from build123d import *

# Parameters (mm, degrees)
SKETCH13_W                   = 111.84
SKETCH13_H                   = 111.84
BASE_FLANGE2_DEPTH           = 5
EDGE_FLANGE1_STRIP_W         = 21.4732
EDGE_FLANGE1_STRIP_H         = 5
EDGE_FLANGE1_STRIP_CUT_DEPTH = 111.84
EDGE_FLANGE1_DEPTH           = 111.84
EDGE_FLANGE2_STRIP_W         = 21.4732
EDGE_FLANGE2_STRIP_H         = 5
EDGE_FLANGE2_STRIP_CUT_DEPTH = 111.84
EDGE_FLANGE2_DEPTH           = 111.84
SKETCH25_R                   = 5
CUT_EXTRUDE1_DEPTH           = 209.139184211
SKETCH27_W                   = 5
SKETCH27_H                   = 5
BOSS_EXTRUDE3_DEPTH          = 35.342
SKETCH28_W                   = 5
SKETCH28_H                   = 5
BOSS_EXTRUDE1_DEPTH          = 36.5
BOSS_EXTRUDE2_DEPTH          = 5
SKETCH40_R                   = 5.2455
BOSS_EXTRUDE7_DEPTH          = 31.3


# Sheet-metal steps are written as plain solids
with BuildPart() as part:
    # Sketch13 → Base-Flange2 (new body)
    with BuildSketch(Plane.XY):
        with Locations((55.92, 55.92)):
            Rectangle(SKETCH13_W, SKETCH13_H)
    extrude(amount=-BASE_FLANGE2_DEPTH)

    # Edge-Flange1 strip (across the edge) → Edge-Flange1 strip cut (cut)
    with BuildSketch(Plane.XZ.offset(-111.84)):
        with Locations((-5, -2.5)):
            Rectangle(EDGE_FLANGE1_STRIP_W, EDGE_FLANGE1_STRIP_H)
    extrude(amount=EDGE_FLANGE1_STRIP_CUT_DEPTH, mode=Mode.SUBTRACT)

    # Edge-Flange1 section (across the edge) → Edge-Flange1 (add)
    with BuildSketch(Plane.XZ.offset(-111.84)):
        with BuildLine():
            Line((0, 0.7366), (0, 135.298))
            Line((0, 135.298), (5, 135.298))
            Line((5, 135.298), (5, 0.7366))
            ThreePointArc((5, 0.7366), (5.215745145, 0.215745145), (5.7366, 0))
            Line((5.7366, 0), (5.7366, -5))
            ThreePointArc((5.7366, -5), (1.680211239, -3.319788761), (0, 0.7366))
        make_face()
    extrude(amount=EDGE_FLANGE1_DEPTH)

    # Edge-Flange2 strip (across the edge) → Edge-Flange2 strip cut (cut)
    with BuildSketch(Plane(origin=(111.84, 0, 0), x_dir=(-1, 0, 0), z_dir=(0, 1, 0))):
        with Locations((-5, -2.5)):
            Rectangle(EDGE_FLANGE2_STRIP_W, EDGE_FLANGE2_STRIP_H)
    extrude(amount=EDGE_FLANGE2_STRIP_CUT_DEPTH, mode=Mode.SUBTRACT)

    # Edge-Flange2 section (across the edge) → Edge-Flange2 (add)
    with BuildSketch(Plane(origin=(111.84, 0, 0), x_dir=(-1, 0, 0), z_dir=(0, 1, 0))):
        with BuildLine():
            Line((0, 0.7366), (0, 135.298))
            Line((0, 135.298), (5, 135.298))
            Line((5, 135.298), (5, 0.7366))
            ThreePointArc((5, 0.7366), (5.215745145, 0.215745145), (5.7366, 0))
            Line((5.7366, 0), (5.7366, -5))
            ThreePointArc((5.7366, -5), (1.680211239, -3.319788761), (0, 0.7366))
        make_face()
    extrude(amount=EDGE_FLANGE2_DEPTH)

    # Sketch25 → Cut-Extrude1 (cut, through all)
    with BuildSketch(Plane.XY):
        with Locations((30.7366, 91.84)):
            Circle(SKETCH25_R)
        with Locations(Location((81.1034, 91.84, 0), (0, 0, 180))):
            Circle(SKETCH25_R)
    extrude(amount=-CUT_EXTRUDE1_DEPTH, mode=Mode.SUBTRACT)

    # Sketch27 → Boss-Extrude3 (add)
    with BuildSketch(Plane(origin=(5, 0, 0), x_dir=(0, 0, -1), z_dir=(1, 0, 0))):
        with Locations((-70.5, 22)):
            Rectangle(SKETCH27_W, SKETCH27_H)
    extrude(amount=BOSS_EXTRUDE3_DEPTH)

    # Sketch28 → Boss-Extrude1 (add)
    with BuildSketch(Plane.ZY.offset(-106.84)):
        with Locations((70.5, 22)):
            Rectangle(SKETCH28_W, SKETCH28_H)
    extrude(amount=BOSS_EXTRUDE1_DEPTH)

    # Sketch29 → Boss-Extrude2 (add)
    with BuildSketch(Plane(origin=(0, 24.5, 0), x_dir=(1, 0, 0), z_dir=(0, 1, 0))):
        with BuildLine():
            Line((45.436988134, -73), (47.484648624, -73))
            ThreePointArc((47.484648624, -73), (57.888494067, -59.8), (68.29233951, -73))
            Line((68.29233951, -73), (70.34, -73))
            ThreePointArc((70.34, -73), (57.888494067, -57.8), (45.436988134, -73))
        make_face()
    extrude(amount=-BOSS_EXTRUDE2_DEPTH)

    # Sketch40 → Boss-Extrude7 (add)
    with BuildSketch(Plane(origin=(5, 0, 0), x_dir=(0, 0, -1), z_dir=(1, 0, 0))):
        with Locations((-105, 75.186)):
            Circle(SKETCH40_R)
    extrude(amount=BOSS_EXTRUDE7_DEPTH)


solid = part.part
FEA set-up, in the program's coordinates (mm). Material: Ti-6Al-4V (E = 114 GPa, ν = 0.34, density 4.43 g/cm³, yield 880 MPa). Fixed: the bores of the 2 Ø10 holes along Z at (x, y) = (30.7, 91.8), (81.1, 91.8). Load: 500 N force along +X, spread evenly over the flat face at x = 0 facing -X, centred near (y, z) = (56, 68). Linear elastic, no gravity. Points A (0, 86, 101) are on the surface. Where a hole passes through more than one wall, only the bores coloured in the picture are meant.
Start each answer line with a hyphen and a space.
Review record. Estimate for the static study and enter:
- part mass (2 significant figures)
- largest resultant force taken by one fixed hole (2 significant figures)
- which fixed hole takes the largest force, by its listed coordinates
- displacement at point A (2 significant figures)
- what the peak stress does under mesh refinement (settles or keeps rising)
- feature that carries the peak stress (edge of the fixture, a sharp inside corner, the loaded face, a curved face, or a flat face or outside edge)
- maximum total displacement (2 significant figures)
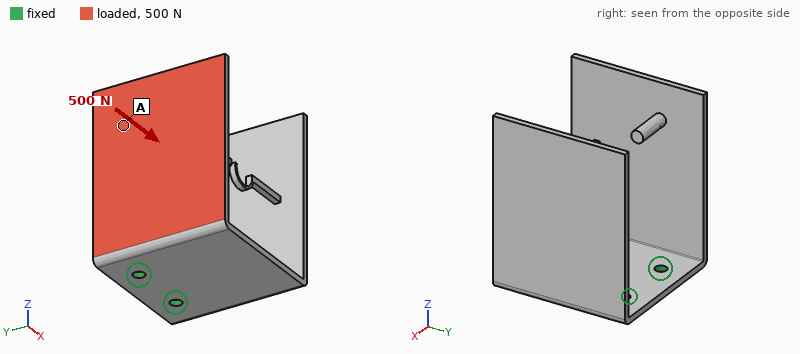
- 960 g
- 530 N
- (30.7, 91.8)
- 1.7 mm
- keeps rising
- edge of the fixture
- 2.5 mm
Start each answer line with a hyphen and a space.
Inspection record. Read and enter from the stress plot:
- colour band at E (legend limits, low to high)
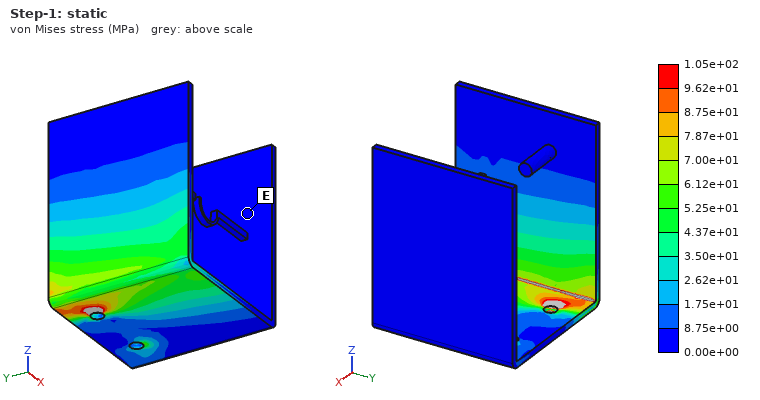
- 0.00e+00 to 8.75e+00 MPa
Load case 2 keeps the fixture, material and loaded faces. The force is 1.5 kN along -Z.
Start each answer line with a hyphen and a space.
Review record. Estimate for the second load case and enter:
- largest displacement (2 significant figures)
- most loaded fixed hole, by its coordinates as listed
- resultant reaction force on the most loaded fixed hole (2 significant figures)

- 2.1 mm
- (30.7, 91.8)
- 1.8 kN
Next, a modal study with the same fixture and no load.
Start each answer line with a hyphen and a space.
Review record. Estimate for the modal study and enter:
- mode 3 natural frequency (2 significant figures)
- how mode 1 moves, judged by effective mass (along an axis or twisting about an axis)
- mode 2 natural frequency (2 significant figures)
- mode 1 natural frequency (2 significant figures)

- 210 Hz
- along X
- 150 Hz
- 140 Hz
